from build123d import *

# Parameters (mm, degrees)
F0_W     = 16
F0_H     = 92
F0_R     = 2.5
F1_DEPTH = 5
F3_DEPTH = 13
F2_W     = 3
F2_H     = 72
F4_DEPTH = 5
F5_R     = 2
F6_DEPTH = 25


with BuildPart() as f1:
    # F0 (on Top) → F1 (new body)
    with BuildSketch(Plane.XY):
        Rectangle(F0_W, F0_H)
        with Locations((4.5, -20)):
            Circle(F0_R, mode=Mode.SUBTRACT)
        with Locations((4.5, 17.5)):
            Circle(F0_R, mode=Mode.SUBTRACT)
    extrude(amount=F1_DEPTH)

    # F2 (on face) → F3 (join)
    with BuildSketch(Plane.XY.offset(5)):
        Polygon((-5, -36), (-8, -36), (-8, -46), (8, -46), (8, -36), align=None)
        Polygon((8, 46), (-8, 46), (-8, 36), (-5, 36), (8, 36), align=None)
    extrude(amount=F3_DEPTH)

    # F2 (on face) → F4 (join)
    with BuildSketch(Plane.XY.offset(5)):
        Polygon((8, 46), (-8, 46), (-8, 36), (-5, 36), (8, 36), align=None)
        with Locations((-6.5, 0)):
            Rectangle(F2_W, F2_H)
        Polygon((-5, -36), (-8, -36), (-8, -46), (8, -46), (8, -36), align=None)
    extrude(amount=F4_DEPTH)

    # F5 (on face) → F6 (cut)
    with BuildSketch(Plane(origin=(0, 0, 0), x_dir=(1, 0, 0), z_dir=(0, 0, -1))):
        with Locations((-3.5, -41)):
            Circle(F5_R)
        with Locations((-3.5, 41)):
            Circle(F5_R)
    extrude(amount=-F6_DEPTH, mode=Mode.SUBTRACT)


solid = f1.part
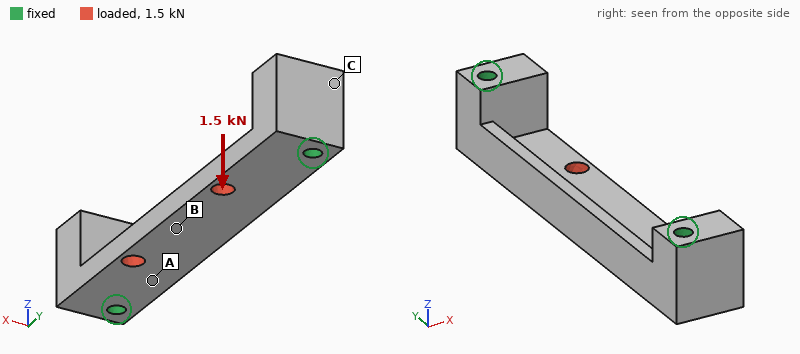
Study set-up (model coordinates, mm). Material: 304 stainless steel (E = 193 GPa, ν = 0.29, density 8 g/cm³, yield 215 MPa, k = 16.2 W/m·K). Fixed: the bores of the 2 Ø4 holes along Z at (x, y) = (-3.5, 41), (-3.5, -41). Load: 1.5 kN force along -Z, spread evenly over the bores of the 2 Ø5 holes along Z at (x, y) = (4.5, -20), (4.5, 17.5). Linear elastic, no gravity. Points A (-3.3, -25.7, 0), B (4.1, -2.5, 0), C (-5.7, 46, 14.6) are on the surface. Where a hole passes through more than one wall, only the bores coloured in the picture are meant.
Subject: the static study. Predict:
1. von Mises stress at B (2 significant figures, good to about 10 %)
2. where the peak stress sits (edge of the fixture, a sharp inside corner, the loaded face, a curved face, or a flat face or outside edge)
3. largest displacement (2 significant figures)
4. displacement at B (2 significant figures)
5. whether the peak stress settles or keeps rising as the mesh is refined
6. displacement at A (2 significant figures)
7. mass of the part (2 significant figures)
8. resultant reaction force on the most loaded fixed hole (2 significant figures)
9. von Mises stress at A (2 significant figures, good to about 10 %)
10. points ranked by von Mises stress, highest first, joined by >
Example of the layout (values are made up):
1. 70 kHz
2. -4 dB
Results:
1. 24 MPa
2. a sharp inside corner
3. 53 µm
4. 43 µm
5. keeps rising
6. 12 µm
7. 96 g
8. 790 N
9. 65 MPa
10. A > B > C
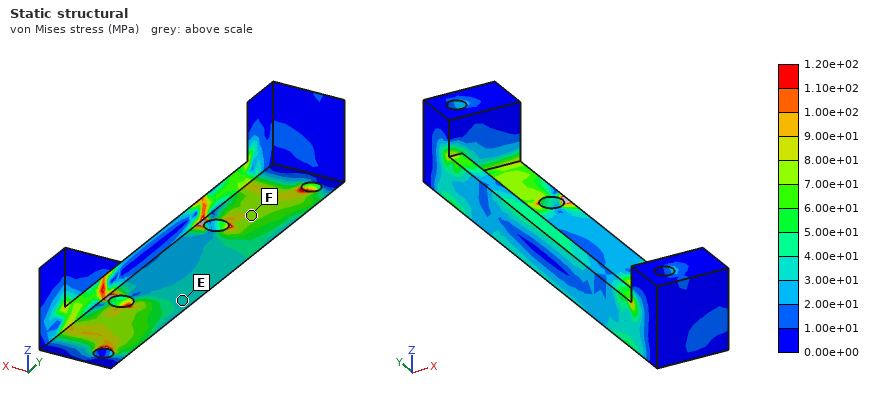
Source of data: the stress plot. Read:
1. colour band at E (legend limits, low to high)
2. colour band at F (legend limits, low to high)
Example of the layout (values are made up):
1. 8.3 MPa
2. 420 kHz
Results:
1. 3.00e+01 to 4.00e+01 MPa
2. 7.00e+01 to 8.00e+01 MPa
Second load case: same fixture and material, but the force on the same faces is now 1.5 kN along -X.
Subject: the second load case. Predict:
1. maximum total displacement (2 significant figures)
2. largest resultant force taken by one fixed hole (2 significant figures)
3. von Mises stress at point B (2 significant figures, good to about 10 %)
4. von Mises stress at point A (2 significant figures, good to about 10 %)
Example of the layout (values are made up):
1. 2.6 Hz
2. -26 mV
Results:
1. 15 µm
2. 800 N
3. 12 MPa
4. 18 MPa
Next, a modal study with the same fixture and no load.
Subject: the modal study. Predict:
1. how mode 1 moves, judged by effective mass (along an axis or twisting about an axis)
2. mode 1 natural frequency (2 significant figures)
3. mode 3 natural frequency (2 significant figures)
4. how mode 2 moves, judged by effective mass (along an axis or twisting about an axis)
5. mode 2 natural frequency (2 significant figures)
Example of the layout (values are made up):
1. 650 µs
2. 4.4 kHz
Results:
1. along Z
2. 5500 Hz
3. 11 kHz
4. along X
5. 7900 Hz
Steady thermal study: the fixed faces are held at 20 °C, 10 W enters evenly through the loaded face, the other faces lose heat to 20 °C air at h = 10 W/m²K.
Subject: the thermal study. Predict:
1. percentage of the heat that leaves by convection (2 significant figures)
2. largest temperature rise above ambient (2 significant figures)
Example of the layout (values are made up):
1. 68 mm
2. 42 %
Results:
1. 18 %
2. 82 K
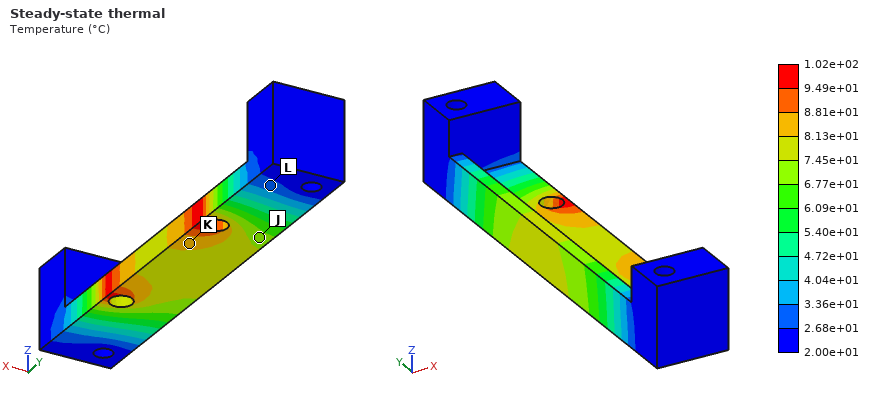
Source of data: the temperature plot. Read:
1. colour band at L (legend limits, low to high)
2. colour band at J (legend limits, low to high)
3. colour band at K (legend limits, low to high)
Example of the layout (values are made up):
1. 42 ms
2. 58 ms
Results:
1. 2.68e+01 to 3.36e+01 °C
2. 6.77e+01 to 7.45e+01 °C
3. 8.13e+01 to 8.81e+01 °C
